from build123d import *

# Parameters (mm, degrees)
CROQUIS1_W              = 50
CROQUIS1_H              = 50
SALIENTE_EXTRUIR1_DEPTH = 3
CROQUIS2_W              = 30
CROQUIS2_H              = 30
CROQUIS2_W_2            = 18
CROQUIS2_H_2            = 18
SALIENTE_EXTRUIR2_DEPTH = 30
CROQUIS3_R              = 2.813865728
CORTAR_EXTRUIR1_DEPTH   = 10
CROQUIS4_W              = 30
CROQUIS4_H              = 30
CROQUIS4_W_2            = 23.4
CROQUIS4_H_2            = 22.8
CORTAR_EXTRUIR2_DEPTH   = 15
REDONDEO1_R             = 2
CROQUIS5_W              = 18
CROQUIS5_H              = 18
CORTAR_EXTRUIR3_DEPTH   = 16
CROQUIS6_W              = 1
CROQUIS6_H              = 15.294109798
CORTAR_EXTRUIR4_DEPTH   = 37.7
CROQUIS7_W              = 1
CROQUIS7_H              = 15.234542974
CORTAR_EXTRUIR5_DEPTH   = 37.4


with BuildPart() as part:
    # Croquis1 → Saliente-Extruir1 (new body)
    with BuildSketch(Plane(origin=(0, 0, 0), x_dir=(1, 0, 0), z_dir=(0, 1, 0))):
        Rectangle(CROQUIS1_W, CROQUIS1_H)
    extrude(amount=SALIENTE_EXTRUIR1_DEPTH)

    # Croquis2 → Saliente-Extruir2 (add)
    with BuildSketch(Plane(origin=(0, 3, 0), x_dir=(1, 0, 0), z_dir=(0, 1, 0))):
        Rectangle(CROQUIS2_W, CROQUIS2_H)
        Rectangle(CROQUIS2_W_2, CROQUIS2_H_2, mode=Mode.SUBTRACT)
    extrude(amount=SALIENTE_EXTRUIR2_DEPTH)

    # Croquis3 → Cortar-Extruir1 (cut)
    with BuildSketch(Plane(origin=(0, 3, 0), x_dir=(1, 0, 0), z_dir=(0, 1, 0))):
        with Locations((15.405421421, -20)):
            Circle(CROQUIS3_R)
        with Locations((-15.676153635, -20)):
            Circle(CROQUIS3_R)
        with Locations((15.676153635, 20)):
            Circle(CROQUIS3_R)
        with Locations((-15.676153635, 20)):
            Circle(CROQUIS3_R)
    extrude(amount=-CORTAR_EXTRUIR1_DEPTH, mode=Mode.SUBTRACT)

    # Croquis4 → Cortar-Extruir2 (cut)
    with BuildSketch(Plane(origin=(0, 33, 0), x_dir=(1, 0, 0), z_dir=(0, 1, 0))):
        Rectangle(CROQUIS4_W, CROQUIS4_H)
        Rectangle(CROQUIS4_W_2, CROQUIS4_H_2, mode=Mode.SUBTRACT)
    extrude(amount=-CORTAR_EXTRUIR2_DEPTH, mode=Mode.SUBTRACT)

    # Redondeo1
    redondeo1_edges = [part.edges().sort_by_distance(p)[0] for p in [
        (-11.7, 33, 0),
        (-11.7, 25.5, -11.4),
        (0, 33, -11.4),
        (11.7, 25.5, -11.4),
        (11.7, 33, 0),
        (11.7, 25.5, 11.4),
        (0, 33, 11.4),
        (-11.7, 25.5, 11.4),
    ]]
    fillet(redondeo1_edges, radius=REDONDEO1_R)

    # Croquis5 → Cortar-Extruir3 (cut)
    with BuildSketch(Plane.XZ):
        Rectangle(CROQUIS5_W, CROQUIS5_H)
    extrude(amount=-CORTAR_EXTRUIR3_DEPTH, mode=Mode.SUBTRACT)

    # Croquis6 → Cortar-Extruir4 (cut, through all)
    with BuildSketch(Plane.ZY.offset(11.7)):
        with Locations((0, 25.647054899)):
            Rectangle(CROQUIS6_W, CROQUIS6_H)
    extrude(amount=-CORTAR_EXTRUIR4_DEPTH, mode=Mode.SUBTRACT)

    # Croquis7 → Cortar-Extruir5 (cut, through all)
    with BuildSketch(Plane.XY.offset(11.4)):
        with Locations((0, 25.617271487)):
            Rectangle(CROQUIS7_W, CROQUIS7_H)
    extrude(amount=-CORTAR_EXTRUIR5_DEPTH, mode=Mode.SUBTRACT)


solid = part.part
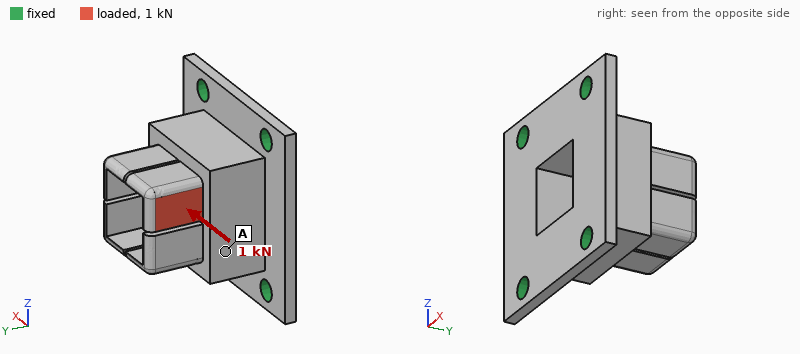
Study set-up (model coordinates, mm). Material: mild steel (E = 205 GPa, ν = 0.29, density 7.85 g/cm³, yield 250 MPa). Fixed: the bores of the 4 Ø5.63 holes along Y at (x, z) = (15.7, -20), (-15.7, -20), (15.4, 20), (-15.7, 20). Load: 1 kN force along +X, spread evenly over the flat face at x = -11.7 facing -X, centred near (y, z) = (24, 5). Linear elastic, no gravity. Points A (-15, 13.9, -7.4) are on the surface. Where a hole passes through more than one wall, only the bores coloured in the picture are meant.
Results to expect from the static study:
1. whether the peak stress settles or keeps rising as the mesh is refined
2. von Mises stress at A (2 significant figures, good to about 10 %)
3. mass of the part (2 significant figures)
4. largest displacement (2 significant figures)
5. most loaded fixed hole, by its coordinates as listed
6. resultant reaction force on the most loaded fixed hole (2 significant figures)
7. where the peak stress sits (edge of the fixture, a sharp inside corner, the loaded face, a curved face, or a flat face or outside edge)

keeps rising
22 MPa
140 g
55 µm
(15.4, 20)
690 N
a sharp inside corner
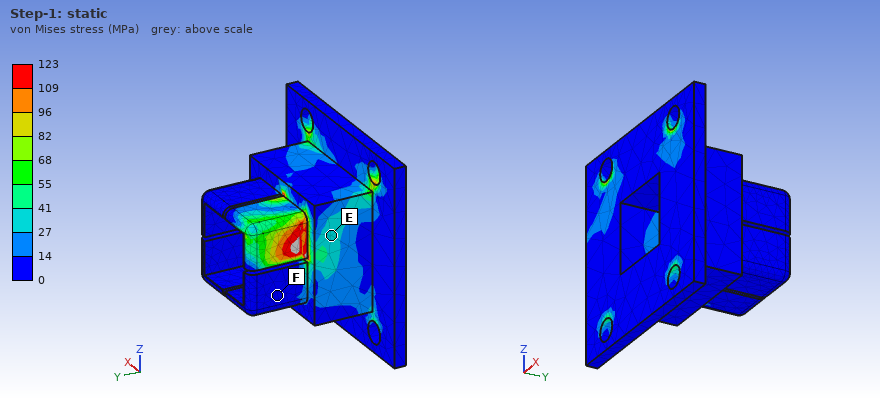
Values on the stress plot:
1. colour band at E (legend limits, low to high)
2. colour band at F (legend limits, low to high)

27 to 41 MPa
0 to 14 MPa
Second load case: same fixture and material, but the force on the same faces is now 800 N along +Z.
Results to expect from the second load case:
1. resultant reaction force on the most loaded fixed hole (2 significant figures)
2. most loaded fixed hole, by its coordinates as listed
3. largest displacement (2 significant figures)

560 N
(-15.7, -20)
22 µm
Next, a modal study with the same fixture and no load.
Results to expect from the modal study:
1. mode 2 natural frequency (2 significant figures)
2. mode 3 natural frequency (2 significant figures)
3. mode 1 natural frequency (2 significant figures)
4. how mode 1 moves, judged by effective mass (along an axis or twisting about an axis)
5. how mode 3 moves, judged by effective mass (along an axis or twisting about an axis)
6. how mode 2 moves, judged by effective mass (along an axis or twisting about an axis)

11 kHz
12 kHz
9300 Hz
along X
along Y
along Z
